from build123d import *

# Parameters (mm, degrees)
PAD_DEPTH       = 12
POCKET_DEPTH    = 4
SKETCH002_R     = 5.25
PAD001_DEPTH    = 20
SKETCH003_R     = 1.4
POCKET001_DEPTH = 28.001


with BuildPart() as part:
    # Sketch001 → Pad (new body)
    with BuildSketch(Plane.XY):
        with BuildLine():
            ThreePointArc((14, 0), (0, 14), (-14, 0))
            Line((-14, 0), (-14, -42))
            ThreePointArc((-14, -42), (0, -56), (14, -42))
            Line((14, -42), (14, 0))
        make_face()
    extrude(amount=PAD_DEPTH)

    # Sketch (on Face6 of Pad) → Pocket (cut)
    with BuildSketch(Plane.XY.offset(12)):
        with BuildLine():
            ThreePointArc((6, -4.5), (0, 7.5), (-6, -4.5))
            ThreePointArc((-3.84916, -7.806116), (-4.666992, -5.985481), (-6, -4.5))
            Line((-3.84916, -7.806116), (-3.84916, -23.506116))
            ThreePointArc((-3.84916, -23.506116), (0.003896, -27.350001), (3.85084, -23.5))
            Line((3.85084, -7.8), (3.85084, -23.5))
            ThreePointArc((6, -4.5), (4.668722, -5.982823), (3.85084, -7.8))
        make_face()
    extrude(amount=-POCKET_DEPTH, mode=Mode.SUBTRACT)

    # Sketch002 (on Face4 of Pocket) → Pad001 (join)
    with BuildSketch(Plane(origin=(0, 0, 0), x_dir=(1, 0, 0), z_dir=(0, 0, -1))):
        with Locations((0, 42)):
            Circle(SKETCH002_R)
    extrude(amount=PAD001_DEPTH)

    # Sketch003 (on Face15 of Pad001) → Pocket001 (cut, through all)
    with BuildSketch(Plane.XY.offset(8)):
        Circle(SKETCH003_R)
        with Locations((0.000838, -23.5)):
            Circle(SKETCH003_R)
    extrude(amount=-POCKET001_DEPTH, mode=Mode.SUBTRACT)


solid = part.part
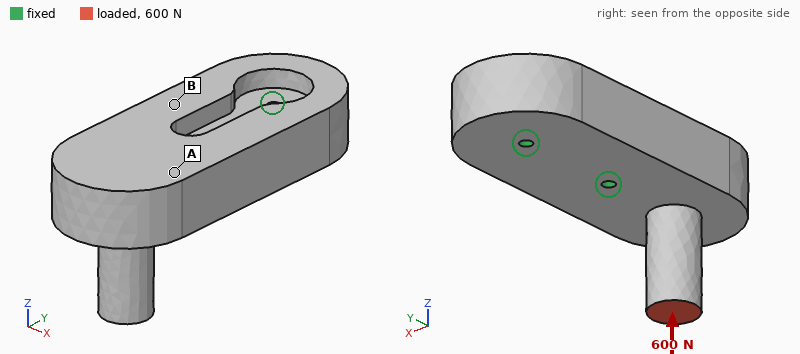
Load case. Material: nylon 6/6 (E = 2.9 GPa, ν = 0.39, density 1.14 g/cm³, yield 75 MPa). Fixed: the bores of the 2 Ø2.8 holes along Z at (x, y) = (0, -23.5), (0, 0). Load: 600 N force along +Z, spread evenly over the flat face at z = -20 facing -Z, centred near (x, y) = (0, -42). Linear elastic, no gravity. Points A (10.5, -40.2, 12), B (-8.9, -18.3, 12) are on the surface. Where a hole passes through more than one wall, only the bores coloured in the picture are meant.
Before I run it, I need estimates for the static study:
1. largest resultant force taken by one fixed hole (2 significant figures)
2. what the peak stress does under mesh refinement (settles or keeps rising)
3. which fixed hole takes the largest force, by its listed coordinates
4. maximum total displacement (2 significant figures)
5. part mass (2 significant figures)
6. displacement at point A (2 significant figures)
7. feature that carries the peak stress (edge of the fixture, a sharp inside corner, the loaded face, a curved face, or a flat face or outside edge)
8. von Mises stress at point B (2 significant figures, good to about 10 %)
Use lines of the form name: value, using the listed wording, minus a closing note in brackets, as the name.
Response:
largest resultant force taken by one fixed hole: 920 N
what the peak stress does under mesh refinement: keeps rising
which fixed hole takes the largest force, by its listed coordinates: (0, -23.5)
maximum total displacement: 0.65 mm
part mass: 25 g
displacement at point A: 0.30 mm
feature that carries the peak stress: edge of the fixture
von Mises stress at point B: 11 MPa
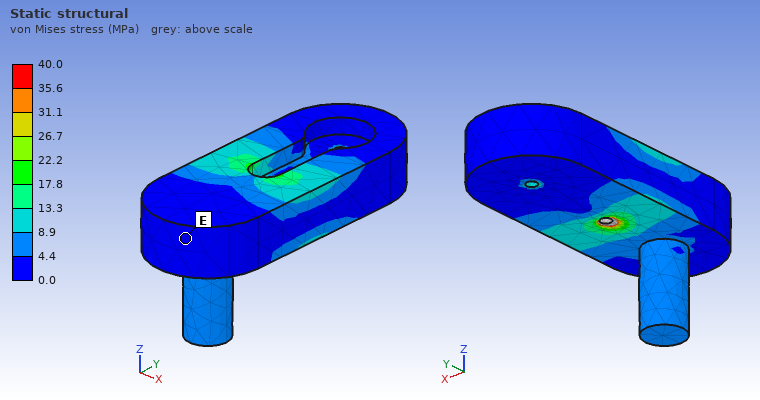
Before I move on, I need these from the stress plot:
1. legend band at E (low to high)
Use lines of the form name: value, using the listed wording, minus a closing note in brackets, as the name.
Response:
legend band at E: 0.0 to 4.4 MPa
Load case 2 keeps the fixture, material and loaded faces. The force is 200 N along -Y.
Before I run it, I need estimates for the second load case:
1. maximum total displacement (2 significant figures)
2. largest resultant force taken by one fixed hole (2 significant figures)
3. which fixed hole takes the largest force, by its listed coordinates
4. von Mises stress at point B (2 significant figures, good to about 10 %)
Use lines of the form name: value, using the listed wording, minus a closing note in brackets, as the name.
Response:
maximum total displacement: 0.82 mm
largest resultant force taken by one fixed hole: 280 N
which fixed hole takes the largest force, by its listed coordinates: (0, -23.5)
von Mises stress at point B: 4.9 MPa
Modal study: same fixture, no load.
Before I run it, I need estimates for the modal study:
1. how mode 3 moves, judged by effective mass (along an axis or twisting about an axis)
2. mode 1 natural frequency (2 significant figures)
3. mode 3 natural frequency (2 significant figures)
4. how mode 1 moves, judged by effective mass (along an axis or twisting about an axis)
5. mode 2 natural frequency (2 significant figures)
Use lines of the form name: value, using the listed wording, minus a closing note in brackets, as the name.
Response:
how mode 3 moves, judged by effective mass: along X
mode 1 natural frequency: 1800 Hz
mode 3 natural frequency: 3000 Hz
how mode 1 moves, judged by effective mass: along Z
mode 2 natural frequency: 2400 Hz
